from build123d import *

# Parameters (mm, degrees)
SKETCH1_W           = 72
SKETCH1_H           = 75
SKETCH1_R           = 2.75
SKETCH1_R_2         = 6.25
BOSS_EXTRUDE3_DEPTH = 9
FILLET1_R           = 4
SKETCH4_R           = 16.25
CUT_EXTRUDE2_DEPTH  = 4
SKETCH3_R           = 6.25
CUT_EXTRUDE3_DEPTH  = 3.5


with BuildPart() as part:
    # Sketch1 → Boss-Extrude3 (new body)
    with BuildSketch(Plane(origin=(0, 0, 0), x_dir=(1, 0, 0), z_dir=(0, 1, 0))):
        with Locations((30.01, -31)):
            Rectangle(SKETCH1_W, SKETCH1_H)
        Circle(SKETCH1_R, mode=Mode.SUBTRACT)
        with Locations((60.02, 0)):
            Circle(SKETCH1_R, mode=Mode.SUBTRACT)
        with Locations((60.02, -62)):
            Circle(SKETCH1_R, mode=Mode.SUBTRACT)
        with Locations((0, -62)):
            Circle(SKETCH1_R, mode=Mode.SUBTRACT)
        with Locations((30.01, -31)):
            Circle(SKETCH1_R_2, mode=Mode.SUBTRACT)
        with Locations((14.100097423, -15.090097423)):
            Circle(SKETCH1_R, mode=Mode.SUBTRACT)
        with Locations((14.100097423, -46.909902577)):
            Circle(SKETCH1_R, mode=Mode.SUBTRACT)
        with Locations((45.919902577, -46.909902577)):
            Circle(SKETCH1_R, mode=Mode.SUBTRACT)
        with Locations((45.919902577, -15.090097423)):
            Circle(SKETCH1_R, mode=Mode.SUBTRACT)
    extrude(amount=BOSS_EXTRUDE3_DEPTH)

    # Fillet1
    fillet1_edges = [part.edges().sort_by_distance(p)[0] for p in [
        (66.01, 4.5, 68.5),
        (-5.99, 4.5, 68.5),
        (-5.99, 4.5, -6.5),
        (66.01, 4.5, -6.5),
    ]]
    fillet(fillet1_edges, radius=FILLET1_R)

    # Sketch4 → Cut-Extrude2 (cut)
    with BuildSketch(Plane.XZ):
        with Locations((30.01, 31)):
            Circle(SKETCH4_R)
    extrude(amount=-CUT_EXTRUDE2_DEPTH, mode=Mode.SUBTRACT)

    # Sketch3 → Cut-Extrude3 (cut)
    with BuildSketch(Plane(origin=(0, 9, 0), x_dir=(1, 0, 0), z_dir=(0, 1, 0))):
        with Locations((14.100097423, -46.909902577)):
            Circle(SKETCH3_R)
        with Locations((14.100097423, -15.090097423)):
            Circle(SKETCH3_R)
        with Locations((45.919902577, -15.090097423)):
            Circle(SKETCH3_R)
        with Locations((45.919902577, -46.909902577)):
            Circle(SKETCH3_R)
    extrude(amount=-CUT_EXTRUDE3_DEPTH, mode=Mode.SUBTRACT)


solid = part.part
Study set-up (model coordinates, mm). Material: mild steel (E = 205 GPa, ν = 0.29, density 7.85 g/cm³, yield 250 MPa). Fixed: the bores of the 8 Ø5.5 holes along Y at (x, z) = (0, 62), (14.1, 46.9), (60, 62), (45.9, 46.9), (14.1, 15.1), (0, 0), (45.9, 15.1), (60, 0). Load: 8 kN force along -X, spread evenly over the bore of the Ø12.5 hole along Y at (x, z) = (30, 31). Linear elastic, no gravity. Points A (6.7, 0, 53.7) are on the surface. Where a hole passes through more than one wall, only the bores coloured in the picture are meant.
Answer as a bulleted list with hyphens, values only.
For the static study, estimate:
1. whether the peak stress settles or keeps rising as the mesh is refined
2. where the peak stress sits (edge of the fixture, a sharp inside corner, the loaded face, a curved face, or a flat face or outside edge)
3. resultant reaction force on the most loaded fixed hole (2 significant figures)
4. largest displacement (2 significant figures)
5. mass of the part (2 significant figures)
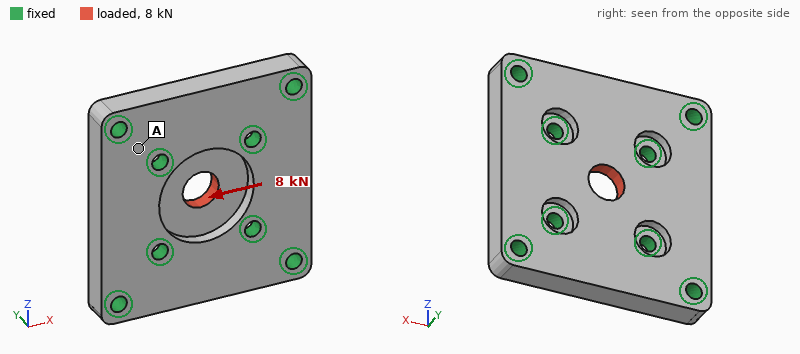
- keeps rising
- edge of the fixture
- 1.7 kN
- 3.9 µm
- 330 g
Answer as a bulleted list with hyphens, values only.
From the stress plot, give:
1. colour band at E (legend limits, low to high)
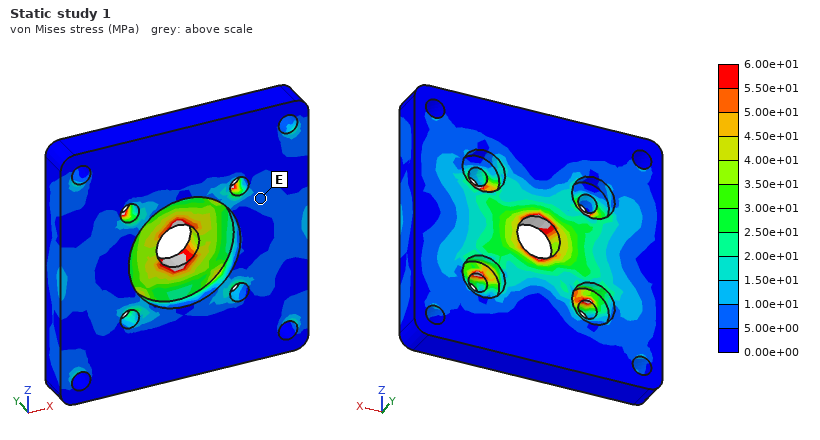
- 5.00e+00 to 1.00e+01 MPa
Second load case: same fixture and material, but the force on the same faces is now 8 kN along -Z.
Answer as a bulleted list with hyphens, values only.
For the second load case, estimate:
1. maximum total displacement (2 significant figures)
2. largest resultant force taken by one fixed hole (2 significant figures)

- 3.9 µm
- 1.7 kN
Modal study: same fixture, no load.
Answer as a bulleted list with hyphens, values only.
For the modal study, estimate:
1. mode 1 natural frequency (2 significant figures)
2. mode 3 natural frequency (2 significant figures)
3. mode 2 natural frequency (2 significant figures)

- 16 kHz
- 17 kHz
- 17 kHz
